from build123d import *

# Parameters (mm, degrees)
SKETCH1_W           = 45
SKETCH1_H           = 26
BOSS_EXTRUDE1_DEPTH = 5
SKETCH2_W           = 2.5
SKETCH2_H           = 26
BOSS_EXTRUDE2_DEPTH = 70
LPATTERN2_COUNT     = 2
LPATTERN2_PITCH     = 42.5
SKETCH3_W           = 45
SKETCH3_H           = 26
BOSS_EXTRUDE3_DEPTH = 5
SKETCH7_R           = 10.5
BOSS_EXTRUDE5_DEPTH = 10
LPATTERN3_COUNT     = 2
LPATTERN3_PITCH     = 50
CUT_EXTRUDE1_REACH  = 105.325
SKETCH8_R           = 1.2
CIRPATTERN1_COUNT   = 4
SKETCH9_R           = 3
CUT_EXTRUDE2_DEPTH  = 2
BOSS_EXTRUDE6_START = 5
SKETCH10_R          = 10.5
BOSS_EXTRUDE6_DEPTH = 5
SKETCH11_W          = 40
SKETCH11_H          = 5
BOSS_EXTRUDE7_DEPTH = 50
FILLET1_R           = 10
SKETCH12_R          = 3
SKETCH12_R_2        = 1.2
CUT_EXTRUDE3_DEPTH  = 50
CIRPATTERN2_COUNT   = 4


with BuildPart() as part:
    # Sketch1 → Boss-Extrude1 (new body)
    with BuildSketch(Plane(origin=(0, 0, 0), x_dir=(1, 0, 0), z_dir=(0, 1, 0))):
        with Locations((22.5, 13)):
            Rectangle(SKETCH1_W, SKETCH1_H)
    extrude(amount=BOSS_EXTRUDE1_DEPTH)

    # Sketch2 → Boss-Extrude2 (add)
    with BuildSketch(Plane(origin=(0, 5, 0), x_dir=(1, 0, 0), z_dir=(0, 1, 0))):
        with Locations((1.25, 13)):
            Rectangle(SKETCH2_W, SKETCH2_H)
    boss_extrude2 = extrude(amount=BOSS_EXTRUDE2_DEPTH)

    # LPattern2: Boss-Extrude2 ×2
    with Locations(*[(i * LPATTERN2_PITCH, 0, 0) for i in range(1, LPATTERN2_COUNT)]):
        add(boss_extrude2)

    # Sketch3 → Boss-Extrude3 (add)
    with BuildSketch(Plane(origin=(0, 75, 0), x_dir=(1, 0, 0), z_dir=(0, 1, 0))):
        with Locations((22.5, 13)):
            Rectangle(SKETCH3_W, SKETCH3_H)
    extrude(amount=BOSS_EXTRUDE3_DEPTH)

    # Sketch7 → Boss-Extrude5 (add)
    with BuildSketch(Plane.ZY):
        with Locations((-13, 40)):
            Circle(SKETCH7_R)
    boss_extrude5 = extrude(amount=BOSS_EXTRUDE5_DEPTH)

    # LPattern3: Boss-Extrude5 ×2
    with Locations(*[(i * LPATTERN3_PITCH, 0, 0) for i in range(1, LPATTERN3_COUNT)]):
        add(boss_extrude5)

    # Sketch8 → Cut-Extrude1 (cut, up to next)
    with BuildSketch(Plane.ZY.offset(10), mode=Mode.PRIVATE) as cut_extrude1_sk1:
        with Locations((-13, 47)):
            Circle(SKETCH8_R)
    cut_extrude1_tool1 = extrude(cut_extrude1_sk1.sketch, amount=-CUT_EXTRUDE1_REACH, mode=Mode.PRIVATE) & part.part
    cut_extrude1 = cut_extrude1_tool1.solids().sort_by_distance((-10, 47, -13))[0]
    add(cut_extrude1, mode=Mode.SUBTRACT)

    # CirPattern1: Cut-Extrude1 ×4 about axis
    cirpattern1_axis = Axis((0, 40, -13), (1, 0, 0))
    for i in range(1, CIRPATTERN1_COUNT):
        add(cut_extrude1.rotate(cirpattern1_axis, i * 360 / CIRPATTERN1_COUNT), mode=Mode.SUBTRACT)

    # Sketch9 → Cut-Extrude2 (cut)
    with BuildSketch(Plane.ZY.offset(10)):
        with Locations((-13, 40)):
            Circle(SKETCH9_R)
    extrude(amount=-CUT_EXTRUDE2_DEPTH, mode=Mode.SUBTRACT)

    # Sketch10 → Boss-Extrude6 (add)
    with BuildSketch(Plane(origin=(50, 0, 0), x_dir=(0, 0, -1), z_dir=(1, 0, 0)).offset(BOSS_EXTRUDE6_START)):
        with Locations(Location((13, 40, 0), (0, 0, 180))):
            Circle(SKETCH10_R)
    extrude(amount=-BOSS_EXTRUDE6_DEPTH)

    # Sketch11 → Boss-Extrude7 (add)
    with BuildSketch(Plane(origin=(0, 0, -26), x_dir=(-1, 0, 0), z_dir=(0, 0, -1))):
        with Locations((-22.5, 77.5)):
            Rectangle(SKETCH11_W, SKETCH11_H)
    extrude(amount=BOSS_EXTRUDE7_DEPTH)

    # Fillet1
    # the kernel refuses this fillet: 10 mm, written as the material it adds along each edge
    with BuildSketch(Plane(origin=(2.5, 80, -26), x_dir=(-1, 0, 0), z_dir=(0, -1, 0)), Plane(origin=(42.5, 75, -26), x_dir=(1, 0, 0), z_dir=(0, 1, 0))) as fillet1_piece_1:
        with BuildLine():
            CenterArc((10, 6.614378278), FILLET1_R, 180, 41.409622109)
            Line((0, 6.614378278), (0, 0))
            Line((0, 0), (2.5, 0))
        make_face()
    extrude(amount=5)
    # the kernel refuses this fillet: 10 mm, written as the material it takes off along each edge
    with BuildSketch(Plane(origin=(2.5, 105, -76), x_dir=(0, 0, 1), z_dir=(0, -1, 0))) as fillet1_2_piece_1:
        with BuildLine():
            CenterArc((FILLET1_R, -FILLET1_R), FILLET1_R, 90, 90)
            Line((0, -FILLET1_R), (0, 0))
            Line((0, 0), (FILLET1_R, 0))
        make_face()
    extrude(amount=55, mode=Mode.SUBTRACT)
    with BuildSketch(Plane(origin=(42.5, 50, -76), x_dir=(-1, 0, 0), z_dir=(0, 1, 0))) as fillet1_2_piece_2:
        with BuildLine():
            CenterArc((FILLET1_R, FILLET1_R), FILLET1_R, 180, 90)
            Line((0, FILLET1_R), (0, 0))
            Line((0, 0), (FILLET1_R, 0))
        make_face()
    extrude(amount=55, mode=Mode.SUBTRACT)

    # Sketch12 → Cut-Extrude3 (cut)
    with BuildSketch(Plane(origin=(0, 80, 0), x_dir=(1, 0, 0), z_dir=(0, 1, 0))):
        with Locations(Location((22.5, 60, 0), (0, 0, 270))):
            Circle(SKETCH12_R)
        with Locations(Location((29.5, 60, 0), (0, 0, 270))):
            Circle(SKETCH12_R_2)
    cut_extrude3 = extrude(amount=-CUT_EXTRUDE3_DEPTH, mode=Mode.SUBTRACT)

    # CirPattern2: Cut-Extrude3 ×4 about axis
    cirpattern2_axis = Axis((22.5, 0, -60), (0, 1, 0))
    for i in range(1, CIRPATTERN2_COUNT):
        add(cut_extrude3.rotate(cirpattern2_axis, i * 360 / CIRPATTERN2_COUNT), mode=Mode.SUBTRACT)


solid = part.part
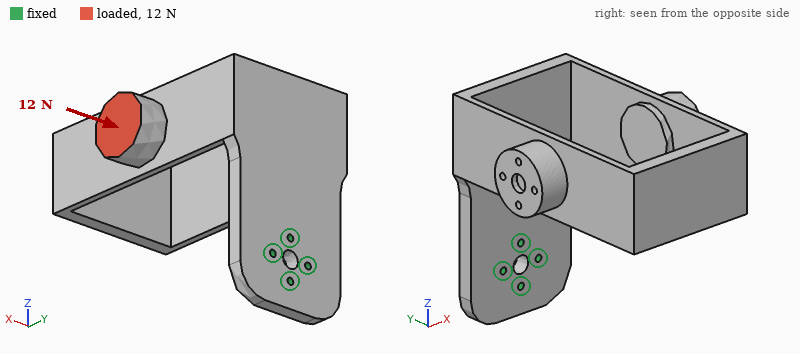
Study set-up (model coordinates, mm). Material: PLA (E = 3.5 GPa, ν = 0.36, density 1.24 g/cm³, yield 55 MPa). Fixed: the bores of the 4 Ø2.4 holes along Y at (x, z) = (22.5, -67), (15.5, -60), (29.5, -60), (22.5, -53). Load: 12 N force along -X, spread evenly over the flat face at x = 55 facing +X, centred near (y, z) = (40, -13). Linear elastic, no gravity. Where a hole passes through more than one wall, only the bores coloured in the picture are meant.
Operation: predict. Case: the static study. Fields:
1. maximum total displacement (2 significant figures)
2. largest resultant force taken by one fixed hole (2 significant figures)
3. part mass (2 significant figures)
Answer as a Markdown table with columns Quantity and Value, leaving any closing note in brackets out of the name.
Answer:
| Quantity | Value |
|---|---|
| maximum total displacement | 1.3 mm |
| largest resultant force taken by one fixed hole | 25 N |
| part mass | 47 g |
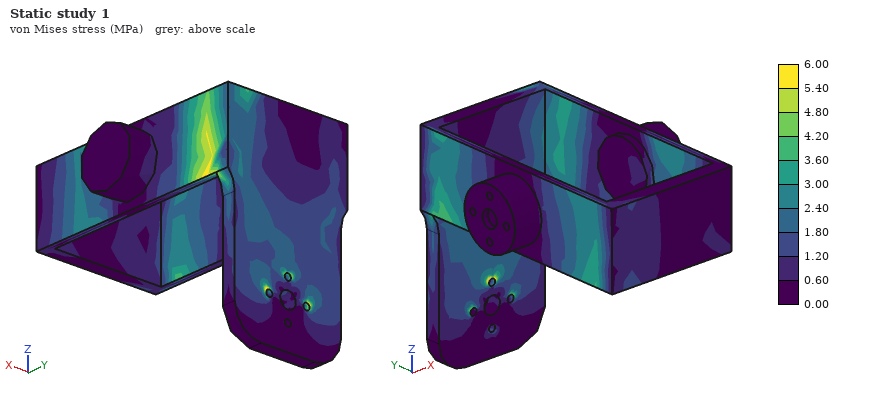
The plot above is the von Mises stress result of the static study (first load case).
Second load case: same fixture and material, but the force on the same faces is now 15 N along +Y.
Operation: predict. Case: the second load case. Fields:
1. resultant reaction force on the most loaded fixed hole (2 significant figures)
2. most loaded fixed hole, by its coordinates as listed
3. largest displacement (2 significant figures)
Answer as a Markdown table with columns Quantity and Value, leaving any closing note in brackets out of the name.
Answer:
| Quantity | Value |
|---|---|
| resultant reaction force on the most loaded fixed hole | 44 N |
| most loaded fixed hole, by its coordinates as listed | (22.5, -53) |
| largest displacement | 1.3 mm |
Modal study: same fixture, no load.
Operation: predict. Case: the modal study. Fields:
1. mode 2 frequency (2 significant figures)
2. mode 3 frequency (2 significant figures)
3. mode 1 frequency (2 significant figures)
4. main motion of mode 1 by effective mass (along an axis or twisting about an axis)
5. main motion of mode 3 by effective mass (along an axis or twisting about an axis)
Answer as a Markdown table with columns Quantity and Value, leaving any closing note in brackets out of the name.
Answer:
| Quantity | Value |
|---|---|
| mode 2 frequency | 100 Hz |
| mode 3 frequency | 390 Hz |
| mode 1 frequency | 94 Hz |
| main motion of mode 1 by effective mass | along X |
| main motion of mode 3 by effective mass | twisting about Y |
